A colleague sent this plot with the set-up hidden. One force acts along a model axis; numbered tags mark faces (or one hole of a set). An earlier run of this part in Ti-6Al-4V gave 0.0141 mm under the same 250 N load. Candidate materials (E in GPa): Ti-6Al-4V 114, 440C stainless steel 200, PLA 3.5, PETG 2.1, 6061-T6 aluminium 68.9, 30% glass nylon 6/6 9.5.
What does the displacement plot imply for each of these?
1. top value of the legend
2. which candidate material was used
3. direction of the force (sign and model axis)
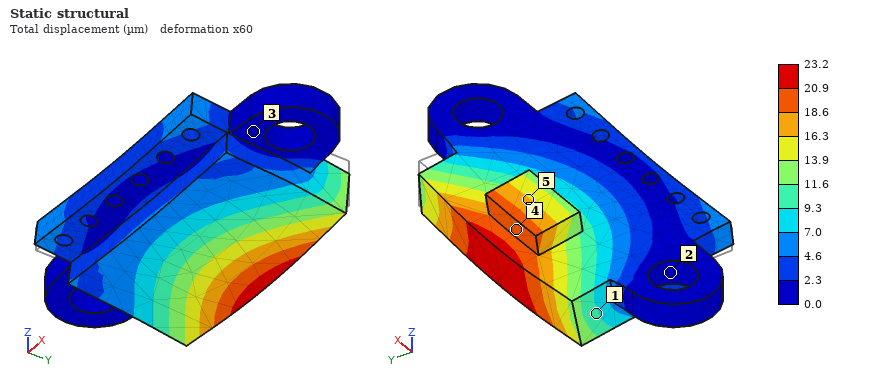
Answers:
23.2 µm
6061-T6 aluminium
-Z
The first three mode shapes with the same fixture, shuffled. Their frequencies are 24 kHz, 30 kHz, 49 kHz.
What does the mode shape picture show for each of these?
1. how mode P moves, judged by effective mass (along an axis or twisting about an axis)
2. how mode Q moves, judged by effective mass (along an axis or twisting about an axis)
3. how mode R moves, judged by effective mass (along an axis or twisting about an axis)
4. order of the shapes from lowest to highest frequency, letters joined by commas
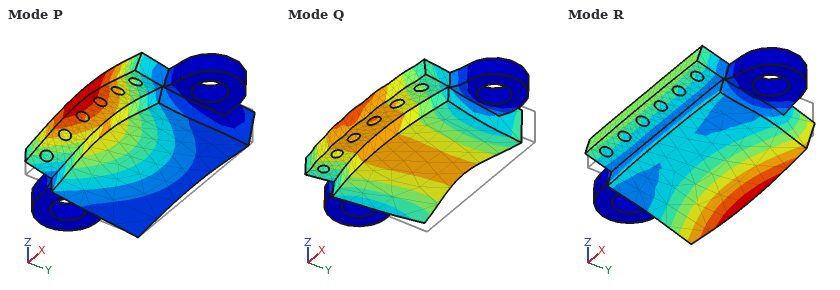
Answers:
along Z
along Y
along Z
R, P, Q
